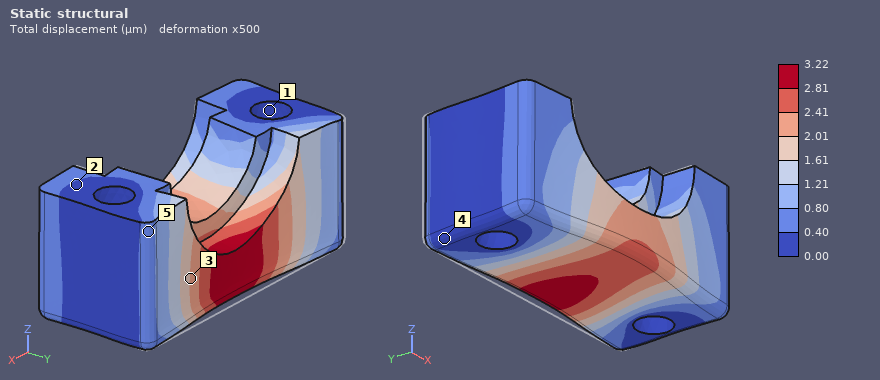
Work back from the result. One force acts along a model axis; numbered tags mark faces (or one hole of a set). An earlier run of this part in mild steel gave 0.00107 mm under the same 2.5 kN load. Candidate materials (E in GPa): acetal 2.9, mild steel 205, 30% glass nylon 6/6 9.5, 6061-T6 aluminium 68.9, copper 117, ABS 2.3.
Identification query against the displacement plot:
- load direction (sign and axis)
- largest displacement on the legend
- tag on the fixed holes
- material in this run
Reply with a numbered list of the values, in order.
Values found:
1. -Y
2. 3.22 µm
3. 1
4. 6061-T6 aluminium
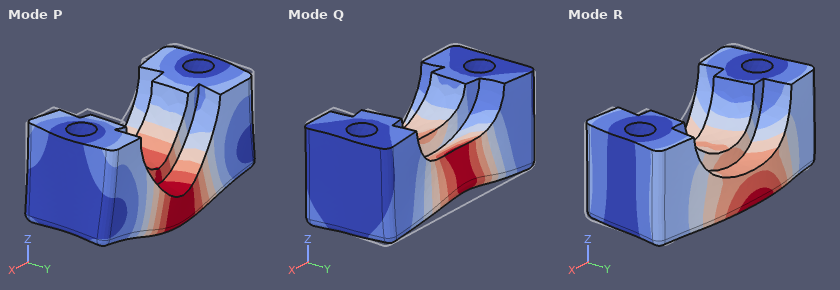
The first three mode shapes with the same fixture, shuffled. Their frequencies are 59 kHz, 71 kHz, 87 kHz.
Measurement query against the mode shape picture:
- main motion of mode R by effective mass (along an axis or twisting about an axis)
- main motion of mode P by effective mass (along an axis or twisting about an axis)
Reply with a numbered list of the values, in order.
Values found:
1. along Y
2. along Z
